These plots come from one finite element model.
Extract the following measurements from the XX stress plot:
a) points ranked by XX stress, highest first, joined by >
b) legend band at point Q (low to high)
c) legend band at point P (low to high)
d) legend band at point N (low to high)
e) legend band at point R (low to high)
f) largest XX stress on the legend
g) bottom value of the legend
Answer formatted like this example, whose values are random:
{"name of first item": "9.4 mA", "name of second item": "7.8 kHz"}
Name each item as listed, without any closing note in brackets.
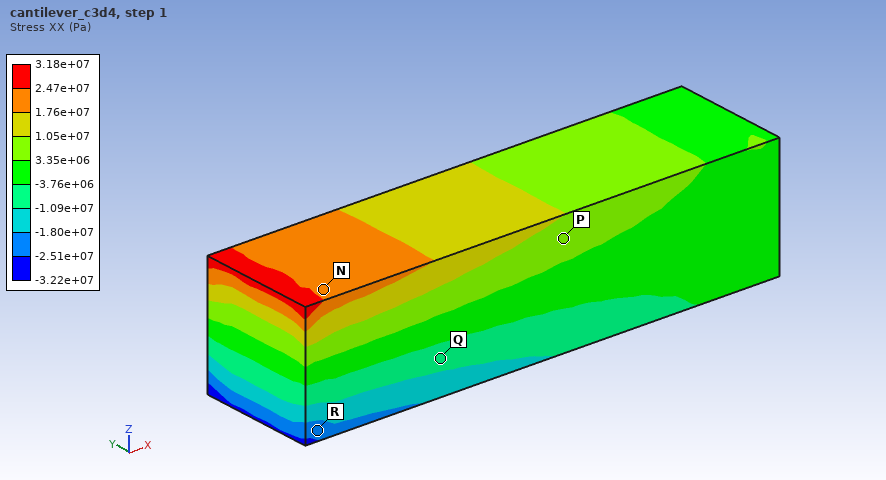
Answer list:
{"points ranked by XX stress, highest first, joined by >": "N > P > Q > R", "legend band at point Q": "-1.09e+07 to -3.76e+06 Pa", "legend band at point P": "3.35e+06 to 1.05e+07 Pa", "legend band at point N": "1.76e+07 to 2.47e+07 Pa", "legend band at point R": "-2.51e+07 to -1.80e+07 Pa", "largest XX stress on the legend": "3.18e+07 Pa", "bottom value of the legend": "-3.22e+07 Pa"}
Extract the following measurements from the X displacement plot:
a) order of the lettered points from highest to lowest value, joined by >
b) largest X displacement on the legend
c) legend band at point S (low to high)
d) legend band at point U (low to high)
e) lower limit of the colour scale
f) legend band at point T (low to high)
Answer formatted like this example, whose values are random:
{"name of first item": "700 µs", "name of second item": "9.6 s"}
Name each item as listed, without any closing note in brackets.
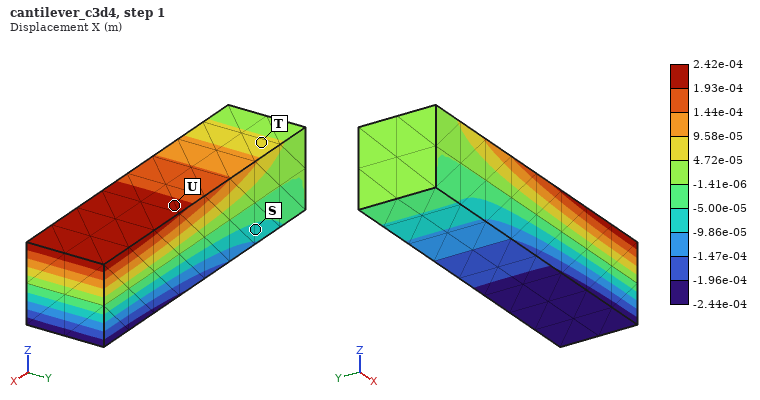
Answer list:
{"order of the lettered points from highest to lowest value, joined by >": "U > T > S", "largest X displacement on the legend": "2.42e-04 m", "legend band at point S": "-9.86e-05 to -5.00e-05 m", "legend band at point U": "1.93e-04 to 2.42e-04 m", "lower limit of the colour scale": "-2.44e-04 m", "legend band at point T": "4.72e-05 to 9.58e-05 m"}
